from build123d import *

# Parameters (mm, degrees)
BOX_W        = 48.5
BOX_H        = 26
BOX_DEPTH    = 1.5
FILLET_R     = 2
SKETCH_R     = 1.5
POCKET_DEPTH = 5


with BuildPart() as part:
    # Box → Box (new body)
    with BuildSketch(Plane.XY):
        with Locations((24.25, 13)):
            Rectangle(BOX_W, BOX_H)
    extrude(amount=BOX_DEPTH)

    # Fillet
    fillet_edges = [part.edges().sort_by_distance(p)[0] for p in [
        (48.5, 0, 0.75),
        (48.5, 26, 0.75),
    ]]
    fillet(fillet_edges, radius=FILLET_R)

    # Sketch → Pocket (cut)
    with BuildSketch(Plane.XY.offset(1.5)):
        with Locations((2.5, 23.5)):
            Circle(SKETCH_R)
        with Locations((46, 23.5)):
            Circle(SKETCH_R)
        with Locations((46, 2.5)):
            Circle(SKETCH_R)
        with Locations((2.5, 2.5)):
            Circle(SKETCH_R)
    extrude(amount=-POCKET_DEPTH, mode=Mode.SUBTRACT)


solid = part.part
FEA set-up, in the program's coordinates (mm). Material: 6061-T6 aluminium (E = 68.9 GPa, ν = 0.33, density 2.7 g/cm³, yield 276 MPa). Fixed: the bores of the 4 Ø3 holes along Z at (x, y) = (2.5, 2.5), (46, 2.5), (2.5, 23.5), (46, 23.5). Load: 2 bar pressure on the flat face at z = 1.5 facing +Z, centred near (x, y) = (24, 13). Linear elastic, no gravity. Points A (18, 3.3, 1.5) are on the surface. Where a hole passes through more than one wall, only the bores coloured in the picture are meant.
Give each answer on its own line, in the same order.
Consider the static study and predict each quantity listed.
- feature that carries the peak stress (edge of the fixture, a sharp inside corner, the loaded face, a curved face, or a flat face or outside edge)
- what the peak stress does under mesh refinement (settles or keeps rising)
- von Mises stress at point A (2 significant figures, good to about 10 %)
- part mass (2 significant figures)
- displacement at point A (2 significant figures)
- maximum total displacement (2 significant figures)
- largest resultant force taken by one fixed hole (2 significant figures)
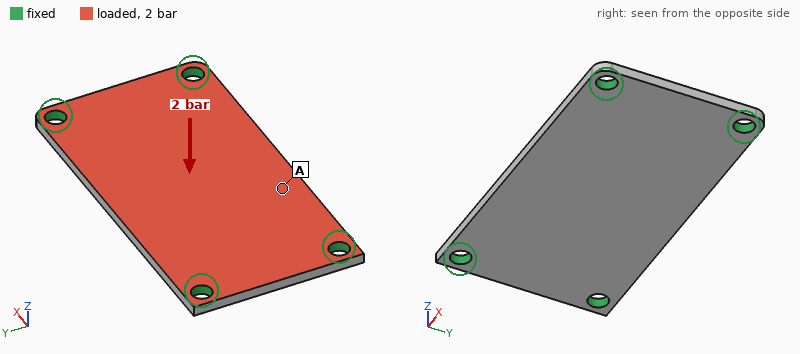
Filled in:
edge of the fixture
keeps rising
33 MPa
5.0 g
0.084 mm
0.10 mm
62 N
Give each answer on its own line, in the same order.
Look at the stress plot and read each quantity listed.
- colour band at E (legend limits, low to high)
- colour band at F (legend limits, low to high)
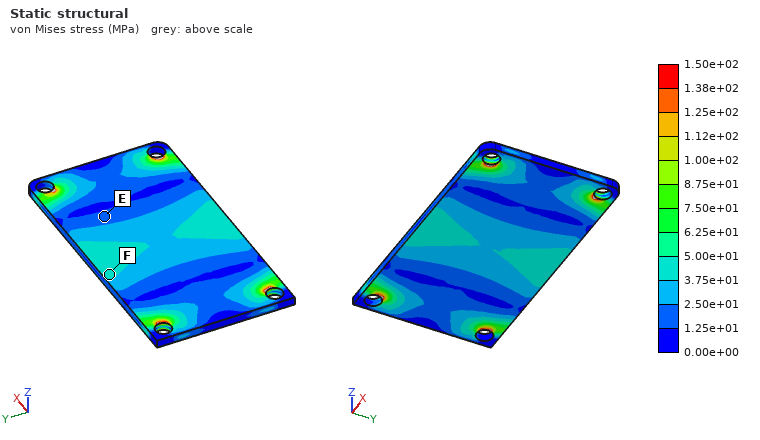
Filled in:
1.25e+01 to 2.50e+01 MPa
3.75e+01 to 5.00e+01 MPa
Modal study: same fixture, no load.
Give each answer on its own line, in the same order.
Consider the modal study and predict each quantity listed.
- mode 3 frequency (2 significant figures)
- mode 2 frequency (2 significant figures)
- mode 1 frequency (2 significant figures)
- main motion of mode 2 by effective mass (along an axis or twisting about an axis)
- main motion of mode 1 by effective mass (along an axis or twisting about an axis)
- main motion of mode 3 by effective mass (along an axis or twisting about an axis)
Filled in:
11 kHz
6500 Hz
4000 Hz
twisting about X
along Z
twisting about Y
